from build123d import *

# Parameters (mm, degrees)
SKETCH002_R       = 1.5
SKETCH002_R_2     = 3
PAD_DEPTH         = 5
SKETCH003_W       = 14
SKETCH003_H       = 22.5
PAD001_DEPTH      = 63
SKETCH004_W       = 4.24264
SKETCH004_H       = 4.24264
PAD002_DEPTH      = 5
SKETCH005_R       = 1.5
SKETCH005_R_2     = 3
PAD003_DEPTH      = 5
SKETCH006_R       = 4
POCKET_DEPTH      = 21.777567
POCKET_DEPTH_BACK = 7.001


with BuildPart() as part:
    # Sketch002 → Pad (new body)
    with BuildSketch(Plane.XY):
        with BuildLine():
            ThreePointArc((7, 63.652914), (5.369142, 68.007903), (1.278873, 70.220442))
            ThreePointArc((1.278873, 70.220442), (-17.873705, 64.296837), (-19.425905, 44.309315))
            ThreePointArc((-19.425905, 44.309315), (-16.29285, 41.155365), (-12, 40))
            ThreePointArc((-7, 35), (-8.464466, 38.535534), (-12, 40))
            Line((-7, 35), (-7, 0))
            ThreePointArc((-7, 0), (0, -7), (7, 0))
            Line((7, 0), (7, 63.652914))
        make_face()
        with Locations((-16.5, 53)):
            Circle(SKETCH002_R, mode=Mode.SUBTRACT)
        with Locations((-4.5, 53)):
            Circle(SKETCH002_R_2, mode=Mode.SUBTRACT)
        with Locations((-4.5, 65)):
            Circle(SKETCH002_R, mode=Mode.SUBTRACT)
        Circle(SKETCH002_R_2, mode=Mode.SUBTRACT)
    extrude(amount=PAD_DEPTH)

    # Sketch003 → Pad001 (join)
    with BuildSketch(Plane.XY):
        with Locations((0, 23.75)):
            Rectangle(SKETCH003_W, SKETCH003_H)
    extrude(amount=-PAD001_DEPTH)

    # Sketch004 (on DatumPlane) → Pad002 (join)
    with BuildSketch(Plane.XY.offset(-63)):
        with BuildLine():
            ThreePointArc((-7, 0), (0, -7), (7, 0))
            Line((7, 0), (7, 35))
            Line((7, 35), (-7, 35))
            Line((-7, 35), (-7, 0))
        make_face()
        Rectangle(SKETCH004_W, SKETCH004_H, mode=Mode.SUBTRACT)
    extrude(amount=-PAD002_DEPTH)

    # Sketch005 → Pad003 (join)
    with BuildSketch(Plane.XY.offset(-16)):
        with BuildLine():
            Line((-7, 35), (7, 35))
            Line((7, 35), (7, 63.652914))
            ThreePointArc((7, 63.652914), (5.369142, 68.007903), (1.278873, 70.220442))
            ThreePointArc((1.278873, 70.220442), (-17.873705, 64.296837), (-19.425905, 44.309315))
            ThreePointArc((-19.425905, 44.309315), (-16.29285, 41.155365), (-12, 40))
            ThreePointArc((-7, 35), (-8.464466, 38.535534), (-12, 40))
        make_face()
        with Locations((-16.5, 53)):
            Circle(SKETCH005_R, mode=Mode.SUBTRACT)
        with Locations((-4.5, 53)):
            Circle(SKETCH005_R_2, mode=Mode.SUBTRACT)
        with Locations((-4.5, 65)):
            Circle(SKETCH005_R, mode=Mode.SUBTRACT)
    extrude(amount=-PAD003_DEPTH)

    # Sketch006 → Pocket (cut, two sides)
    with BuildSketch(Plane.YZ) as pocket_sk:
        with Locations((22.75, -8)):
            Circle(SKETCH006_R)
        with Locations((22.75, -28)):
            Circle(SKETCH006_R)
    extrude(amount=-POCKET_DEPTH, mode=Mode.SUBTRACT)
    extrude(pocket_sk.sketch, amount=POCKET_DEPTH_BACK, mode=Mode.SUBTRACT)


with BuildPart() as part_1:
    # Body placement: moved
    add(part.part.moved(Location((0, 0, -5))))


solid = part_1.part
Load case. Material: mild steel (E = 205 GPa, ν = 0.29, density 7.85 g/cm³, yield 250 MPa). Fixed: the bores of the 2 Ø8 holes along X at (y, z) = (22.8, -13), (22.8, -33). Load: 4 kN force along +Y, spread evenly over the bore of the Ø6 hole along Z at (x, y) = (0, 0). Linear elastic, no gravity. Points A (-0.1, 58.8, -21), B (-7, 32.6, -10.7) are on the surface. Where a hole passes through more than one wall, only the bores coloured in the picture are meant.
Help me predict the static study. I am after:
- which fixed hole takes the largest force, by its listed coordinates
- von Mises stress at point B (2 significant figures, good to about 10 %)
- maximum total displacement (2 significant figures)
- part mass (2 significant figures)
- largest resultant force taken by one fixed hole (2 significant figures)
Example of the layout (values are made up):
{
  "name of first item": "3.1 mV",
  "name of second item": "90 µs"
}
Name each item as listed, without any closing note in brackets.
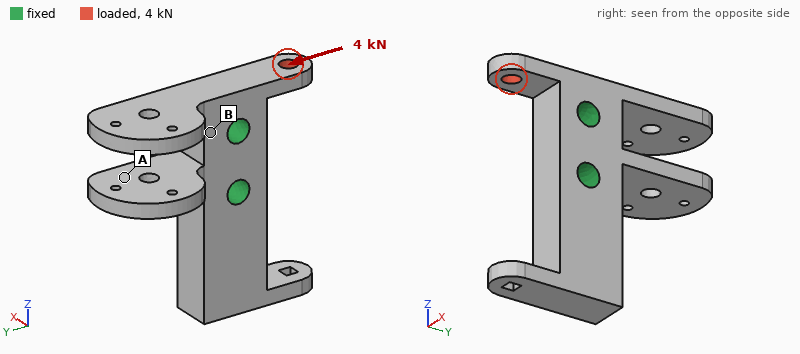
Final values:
{
  "which fixed hole takes the largest force, by its listed coordinates": "(22.8, -13)",
  "von Mises stress at point B": "13 MPa",
  "maximum total displacement": "17 µm",
  "part mass": "250 g",
  "largest resultant force taken by one fixed hole": "4.7 kN"
}
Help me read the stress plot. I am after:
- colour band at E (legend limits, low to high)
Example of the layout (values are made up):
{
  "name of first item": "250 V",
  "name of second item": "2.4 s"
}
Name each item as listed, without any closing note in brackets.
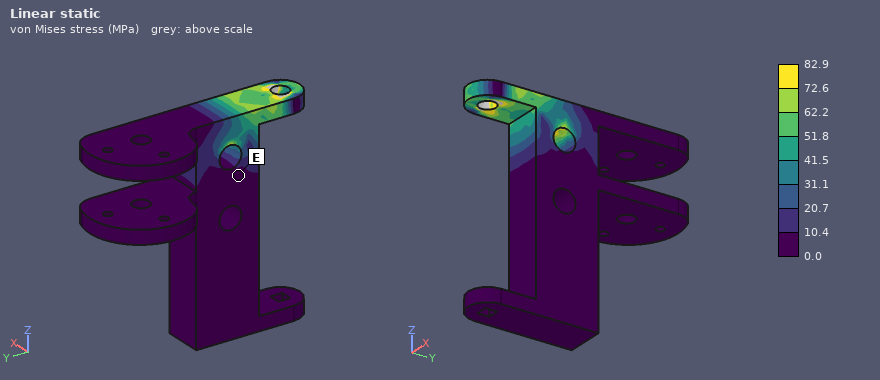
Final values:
{
  "colour band at E": "0.0 to 10.4 MPa"
}
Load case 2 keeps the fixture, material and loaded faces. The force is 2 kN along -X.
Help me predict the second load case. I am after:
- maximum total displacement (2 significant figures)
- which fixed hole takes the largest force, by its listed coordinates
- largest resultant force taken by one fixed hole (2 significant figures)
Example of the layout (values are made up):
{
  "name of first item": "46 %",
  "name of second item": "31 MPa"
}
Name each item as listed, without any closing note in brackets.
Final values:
{
  "maximum total displacement": "48 µm",
  "which fixed hole takes the largest force, by its listed coordinates": "(22.8, -13)",
  "largest resultant force taken by one fixed hole": "2.1 kN"
}
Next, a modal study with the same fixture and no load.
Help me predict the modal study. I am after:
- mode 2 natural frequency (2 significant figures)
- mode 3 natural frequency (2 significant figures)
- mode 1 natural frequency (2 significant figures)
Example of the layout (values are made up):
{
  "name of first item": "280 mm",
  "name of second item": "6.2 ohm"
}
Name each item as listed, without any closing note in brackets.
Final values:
{
  "mode 2 natural frequency": "2500 Hz",
  "mode 3 natural frequency": "4400 Hz",
  "mode 1 natural frequency": "2300 Hz"
}
